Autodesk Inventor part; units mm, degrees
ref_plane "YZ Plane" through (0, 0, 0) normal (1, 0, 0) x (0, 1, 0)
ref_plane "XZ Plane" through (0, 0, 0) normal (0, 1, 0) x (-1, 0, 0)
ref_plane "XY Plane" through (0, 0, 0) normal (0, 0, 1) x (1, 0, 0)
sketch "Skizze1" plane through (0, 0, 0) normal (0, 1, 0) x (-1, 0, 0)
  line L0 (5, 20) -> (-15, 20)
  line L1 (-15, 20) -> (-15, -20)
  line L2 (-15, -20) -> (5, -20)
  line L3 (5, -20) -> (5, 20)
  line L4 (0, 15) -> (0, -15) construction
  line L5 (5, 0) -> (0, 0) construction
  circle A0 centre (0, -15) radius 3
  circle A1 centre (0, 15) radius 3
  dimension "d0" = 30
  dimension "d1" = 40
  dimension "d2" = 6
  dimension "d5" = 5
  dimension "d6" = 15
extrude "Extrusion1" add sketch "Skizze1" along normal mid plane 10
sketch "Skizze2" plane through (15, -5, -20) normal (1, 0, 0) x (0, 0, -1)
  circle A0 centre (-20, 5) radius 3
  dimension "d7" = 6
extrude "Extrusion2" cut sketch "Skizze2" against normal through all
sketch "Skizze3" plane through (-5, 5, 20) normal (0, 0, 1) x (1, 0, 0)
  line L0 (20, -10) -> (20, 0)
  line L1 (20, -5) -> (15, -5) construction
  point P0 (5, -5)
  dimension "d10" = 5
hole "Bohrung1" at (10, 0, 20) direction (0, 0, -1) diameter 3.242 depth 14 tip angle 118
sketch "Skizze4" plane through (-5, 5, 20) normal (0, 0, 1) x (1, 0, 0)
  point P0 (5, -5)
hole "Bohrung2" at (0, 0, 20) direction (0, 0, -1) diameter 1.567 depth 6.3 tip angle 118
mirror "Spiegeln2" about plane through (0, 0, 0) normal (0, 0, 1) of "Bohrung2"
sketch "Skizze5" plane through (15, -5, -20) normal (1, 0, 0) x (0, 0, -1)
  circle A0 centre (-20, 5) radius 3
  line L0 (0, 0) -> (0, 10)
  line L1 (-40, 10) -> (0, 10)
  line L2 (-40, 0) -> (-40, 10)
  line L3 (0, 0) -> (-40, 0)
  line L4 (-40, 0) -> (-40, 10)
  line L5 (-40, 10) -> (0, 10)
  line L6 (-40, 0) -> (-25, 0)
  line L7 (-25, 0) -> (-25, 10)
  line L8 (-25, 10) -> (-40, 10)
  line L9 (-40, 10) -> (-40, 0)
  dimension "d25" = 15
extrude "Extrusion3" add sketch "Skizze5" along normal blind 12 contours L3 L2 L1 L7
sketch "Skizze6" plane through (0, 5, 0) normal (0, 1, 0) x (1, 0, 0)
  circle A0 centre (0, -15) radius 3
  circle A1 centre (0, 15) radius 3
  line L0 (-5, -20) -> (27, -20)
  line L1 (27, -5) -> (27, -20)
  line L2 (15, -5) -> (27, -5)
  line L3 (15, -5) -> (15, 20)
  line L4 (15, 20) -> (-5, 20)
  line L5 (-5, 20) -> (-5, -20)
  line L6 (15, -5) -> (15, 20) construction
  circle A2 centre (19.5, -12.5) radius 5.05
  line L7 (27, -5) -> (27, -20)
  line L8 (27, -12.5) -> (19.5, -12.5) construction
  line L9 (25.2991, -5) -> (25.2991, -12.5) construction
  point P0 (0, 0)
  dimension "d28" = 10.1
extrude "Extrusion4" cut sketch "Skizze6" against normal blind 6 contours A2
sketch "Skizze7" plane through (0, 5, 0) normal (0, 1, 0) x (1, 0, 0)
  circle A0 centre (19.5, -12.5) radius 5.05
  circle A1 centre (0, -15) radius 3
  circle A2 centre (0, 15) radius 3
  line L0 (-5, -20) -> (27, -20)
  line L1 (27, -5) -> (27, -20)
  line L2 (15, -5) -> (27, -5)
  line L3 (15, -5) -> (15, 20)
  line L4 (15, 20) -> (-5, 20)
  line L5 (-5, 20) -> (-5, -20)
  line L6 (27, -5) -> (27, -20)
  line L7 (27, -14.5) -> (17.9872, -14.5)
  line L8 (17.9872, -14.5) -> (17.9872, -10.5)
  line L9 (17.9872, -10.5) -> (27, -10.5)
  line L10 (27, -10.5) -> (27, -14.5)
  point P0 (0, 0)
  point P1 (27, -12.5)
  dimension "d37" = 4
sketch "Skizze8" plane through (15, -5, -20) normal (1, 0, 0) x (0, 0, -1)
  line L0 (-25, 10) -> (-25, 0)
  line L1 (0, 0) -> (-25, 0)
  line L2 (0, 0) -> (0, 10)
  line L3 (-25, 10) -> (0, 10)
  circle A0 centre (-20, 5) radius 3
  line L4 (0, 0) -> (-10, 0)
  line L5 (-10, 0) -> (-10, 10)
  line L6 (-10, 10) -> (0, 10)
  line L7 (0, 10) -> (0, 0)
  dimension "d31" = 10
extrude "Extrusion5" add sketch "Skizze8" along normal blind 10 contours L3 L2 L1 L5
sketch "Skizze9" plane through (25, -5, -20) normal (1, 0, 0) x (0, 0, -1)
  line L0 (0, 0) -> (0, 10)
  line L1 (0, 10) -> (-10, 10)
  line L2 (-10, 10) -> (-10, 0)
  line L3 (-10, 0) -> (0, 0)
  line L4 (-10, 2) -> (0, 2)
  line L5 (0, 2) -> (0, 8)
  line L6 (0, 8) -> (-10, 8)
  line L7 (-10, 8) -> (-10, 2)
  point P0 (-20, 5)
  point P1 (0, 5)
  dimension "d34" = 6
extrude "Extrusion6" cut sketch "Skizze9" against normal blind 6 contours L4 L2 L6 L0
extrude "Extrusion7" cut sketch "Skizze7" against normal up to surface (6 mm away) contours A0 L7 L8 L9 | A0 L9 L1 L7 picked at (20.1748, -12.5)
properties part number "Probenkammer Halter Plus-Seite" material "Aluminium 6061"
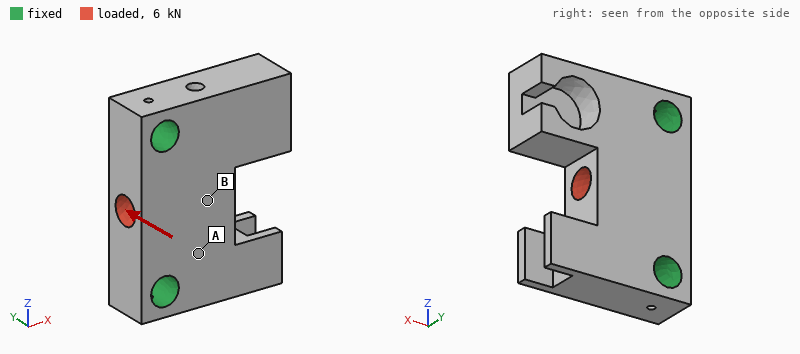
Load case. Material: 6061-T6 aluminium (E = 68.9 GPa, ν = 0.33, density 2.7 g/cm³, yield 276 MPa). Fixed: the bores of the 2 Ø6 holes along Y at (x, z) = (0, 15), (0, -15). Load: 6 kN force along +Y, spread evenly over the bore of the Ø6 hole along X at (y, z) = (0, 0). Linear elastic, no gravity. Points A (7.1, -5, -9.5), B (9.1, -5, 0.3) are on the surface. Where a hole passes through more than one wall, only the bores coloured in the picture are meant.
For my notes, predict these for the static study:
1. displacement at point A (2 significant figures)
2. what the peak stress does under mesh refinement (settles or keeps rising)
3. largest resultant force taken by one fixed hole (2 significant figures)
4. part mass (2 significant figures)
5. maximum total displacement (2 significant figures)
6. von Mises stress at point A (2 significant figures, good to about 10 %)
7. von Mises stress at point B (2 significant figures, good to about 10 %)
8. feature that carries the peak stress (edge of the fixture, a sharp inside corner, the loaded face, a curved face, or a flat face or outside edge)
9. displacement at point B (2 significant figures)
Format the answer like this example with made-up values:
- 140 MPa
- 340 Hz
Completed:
- 12 µm
- keeps rising
- 3.0 kN
- 23 g
- 37 µm
- 24 MPa
- 79 MPa
- edge of the fixture
- 24 µm
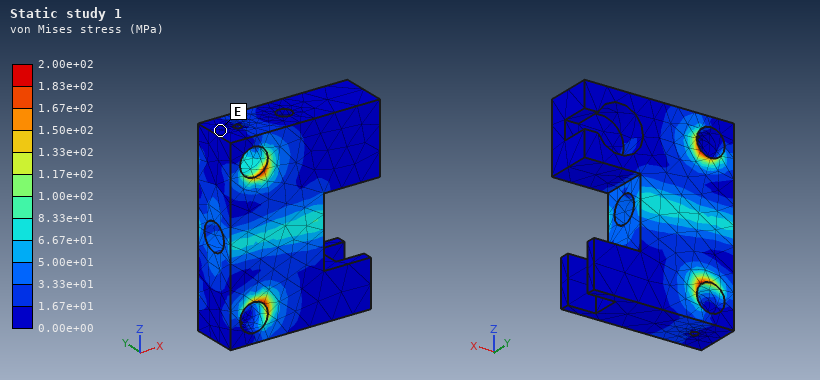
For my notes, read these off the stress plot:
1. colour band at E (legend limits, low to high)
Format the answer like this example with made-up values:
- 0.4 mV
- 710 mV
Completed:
- 0.00e+00 to 1.67e+01 MPa
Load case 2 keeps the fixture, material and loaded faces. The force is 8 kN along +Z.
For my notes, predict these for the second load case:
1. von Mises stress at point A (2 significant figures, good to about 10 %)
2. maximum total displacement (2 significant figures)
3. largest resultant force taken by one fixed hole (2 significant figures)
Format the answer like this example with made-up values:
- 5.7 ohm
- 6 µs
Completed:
- 23 MPa
- 10 µm
- 4.1 kN
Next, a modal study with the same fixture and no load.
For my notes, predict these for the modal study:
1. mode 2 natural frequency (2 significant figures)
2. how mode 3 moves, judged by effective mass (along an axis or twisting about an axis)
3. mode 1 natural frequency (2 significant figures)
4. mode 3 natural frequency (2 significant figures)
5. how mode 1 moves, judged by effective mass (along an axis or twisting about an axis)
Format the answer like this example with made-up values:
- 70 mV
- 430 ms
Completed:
- 18 kHz
- along Z
- 13 kHz
- 19 kHz
- along Y
